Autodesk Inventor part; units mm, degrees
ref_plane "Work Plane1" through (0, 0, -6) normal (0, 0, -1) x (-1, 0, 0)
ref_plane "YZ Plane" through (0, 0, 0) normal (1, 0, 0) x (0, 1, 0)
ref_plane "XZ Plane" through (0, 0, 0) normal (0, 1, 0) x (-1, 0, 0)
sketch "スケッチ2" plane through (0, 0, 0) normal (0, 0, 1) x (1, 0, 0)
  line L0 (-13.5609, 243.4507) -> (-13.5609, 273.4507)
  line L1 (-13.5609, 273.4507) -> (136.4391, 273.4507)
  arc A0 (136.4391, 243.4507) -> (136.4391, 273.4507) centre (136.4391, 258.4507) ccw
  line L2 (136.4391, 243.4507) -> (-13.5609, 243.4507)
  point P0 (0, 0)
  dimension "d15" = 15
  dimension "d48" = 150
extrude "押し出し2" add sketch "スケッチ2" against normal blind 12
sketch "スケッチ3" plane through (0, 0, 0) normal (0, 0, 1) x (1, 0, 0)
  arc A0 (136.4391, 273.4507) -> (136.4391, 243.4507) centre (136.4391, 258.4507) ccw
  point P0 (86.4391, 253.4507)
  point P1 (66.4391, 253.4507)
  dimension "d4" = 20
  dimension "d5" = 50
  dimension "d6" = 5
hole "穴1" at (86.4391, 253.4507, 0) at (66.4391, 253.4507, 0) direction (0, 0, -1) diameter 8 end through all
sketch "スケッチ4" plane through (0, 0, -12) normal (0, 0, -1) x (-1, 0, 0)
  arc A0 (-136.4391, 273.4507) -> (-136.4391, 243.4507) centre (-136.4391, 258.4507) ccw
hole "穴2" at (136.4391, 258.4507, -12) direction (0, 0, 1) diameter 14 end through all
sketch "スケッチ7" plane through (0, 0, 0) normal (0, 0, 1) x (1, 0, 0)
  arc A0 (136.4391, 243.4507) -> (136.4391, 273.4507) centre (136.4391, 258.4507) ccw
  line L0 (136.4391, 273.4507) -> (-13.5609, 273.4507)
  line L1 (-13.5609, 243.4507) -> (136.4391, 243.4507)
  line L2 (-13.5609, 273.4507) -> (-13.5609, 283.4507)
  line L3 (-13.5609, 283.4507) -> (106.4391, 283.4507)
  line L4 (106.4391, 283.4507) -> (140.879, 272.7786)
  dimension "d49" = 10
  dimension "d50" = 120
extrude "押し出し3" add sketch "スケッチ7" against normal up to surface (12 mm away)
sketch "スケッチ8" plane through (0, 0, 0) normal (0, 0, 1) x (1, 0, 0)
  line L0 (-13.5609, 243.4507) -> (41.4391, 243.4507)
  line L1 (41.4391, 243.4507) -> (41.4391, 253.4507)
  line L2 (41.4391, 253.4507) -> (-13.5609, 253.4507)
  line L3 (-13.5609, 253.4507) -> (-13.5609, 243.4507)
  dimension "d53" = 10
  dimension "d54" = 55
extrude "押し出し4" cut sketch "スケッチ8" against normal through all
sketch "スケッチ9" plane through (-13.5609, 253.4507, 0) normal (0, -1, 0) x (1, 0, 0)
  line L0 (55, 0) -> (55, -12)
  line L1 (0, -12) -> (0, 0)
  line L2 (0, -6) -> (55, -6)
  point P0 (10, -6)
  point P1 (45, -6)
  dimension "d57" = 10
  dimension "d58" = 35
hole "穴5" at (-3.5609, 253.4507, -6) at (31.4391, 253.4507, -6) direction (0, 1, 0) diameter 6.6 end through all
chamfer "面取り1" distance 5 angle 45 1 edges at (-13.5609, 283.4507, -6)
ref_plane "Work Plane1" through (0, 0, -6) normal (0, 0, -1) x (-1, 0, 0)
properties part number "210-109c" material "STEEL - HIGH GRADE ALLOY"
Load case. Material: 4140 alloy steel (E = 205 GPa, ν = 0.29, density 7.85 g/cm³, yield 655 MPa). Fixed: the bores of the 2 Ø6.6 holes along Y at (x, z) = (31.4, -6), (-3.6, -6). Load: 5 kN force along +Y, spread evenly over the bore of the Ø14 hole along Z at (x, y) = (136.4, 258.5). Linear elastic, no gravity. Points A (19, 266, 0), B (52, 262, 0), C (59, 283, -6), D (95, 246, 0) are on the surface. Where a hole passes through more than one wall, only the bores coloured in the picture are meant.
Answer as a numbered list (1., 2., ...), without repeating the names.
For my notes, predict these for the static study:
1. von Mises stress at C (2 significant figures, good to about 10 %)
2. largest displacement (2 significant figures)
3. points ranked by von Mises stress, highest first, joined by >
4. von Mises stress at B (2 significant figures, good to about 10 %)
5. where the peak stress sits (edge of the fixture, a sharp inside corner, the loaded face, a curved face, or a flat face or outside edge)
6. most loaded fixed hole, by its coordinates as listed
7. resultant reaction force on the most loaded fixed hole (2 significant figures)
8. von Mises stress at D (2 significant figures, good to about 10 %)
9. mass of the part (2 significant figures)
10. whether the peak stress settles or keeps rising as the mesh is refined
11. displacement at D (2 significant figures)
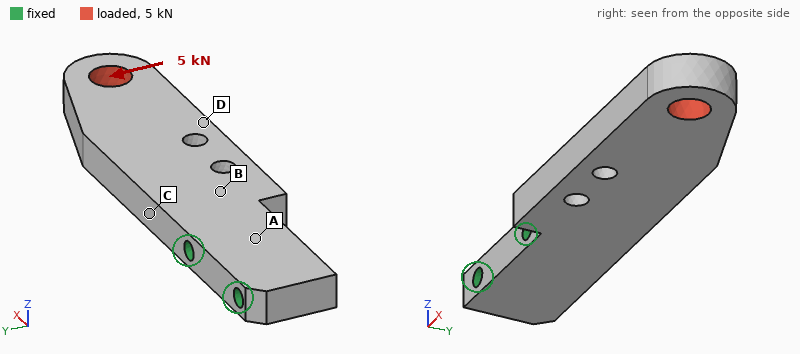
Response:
1. 150 MPa
2. 0.30 mm
3. C > B > D > A
4. 93 MPa
5. edge of the fixture
6. (31.4, -6)
7. 5.2 kN
8. 69 MPa
9. 490 g
10. keeps rising
11. 0.14 mm
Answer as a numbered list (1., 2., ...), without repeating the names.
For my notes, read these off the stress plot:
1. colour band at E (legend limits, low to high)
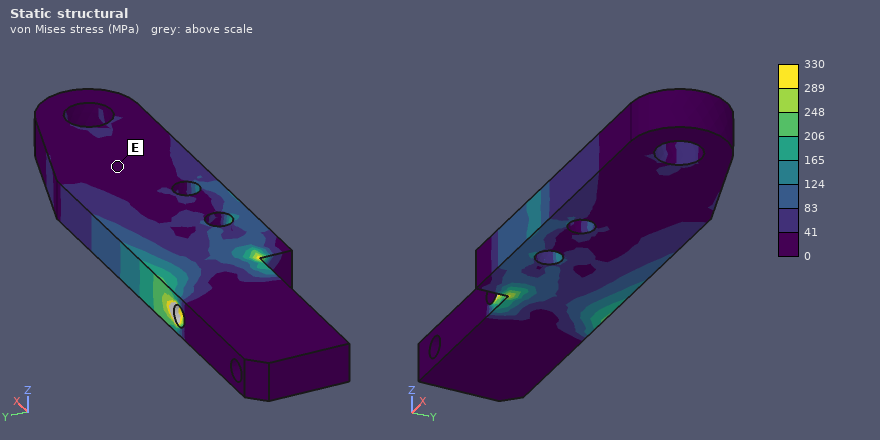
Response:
1. 0 to 41 MPa
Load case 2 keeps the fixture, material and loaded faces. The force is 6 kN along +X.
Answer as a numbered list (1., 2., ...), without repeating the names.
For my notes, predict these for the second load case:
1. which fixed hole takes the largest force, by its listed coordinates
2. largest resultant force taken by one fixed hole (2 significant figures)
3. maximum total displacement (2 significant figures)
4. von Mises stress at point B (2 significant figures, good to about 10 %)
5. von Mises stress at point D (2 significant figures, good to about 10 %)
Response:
1. (31.4, -6)
2. 5.9 kN
3. 38 µm
4. 25 MPa
5. 25 MPa
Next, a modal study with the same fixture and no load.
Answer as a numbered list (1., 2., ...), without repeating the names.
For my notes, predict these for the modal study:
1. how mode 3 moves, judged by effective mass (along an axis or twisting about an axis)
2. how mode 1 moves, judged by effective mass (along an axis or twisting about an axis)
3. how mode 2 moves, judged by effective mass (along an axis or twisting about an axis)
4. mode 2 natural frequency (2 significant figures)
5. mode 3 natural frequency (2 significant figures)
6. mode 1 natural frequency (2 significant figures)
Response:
1. twisting about X
2. along Z
3. along Y
4. 2000 Hz
5. 4000 Hz
6. 760 Hz
